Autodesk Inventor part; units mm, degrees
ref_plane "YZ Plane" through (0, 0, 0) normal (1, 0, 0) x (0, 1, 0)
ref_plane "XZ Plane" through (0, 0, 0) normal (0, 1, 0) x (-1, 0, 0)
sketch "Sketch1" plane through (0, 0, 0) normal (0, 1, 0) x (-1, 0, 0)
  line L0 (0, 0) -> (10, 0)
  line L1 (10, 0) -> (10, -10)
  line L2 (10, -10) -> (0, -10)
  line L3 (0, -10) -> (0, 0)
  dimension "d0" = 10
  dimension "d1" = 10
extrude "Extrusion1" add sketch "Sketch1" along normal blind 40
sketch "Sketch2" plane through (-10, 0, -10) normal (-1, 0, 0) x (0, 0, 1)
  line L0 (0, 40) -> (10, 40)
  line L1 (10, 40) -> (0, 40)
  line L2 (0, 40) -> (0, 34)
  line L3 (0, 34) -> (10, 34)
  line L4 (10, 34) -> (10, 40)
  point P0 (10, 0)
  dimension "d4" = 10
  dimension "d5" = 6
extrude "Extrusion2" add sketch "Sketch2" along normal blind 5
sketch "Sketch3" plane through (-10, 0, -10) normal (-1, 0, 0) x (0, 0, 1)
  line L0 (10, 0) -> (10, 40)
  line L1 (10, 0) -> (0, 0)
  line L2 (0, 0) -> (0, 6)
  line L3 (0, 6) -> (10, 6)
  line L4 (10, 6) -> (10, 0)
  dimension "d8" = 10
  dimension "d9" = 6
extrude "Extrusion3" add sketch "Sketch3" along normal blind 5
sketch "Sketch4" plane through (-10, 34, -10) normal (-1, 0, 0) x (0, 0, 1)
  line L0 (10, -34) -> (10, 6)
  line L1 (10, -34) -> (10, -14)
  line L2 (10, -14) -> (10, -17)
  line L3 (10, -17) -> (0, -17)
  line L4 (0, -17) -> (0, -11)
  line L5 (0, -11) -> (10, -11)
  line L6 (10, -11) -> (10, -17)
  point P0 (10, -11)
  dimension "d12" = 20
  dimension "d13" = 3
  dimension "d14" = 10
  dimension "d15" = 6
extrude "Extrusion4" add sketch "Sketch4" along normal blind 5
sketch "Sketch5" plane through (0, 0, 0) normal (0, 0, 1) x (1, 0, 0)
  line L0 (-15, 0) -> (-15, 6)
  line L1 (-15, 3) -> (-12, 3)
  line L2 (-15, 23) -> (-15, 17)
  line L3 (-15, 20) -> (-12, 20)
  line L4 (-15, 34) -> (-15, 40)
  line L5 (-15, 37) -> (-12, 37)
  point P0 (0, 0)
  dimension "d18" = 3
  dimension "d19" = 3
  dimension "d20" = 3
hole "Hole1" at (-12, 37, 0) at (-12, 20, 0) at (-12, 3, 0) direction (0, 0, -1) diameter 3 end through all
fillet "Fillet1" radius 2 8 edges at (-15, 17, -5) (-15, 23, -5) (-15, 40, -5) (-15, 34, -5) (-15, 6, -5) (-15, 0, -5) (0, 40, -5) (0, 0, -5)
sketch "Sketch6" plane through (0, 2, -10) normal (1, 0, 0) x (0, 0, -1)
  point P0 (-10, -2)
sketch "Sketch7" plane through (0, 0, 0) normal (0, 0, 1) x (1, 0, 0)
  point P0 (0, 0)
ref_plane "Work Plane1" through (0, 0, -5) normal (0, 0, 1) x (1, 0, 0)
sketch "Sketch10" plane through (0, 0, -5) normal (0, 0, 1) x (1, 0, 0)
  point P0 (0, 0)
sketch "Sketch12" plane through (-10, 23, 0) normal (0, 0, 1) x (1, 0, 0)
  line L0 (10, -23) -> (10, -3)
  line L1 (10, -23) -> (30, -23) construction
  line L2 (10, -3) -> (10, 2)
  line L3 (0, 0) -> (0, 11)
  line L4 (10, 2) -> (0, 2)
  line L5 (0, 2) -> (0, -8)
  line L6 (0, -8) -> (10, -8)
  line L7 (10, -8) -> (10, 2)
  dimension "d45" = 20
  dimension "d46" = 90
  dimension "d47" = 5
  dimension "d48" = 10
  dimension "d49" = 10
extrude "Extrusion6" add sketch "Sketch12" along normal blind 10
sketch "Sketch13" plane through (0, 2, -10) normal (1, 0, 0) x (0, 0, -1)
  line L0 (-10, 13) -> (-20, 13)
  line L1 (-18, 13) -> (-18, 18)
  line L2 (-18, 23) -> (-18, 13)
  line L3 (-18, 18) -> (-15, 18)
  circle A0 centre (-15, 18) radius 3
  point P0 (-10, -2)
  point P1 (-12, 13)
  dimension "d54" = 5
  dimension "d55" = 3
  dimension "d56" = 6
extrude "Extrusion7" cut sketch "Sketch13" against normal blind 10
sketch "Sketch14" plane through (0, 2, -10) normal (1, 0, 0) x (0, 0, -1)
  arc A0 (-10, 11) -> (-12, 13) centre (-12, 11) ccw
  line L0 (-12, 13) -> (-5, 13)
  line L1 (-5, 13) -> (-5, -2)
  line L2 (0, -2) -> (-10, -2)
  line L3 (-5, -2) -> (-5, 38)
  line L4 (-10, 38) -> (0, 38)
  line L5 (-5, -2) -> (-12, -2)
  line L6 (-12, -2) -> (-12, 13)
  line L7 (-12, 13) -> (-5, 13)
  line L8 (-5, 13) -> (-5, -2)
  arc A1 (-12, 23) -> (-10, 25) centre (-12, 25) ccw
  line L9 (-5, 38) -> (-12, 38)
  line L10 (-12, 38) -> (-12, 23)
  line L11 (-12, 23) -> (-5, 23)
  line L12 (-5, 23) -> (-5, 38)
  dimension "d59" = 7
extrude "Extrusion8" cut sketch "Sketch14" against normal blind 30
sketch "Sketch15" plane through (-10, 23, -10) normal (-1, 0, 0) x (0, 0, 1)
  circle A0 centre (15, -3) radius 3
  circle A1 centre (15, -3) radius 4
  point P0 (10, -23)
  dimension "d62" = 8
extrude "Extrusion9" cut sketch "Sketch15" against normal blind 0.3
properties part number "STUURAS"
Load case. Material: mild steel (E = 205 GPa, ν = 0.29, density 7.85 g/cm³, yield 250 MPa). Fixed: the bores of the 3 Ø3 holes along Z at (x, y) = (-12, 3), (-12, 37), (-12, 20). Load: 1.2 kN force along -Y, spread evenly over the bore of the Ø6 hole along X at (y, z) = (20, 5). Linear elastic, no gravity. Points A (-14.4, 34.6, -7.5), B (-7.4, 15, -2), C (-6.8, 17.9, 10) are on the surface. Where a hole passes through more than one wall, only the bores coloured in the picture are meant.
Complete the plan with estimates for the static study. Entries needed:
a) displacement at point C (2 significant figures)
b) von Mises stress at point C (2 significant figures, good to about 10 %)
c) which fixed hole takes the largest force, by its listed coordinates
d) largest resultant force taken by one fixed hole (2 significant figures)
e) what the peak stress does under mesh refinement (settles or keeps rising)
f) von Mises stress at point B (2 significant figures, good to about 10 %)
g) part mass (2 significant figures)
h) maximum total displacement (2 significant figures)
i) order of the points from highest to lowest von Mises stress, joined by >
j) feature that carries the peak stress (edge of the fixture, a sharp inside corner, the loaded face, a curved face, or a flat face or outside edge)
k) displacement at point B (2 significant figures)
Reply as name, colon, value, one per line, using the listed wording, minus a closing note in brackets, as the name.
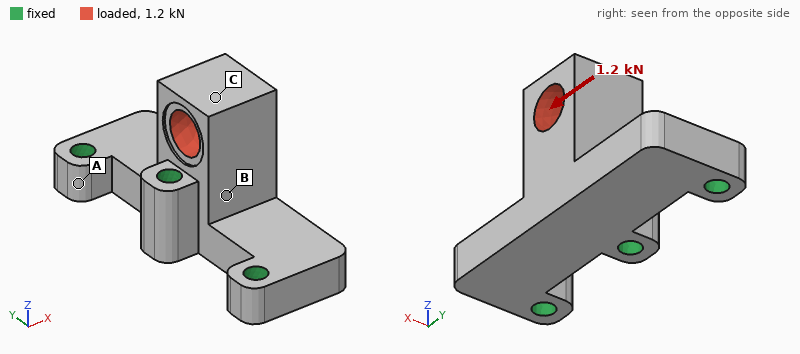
displacement at point C: 16 µm
von Mises stress at point C: 27 MPa
which fixed hole takes the largest force, by its listed coordinates: (-12, 20)
largest resultant force taken by one fixed hole: 910 N
what the peak stress does under mesh refinement: keeps rising
von Mises stress at point B: 68 MPa
part mass: 28 g
maximum total displacement: 18 µm
order of the points from highest to lowest von Mises stress, joined by >: B > C > A
feature that carries the peak stress: edge of the fixture
displacement at point B: 3.7 µm
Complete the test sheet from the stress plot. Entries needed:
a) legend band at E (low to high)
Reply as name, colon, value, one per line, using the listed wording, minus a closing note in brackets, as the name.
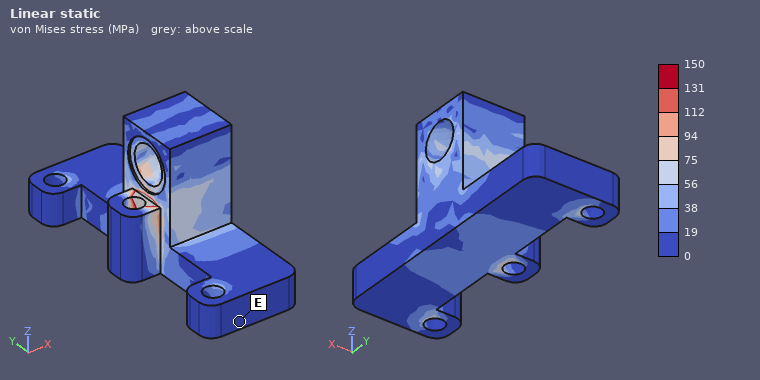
legend band at E: 0 to 19 MPa
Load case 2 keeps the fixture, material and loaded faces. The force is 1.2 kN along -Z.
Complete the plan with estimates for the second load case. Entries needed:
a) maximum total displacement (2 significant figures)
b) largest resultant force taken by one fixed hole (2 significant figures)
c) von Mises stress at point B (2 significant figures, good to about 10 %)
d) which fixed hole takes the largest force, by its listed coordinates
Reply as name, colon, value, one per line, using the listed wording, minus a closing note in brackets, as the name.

maximum total displacement: 5.8 µm
largest resultant force taken by one fixed hole: 1.1 kN
von Mises stress at point B: 21 MPa
which fixed hole takes the largest force, by its listed coordinates: (-12, 20)
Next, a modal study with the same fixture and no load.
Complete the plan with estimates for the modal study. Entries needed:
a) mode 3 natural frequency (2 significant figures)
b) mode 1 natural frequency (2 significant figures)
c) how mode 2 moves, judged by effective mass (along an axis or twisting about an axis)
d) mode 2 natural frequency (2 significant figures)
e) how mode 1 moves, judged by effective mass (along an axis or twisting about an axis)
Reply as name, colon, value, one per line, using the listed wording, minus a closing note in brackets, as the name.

mode 3 natural frequency: 34 kHz
mode 1 natural frequency: 19 kHz
how mode 2 moves, judged by effective mass: along Z
mode 2 natural frequency: 20 kHz
how mode 1 moves, judged by effective mass: along Y
